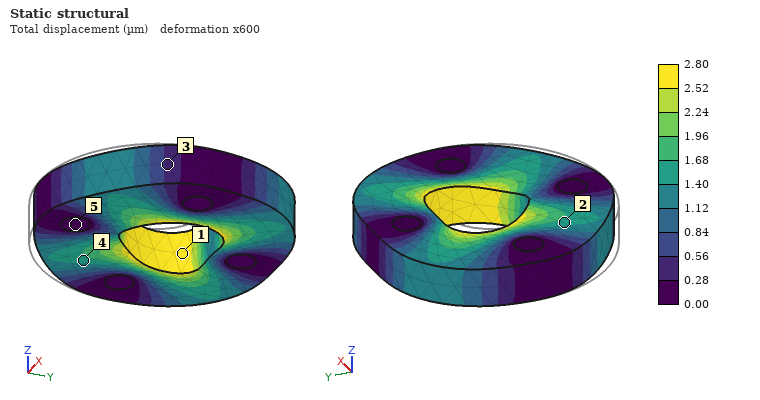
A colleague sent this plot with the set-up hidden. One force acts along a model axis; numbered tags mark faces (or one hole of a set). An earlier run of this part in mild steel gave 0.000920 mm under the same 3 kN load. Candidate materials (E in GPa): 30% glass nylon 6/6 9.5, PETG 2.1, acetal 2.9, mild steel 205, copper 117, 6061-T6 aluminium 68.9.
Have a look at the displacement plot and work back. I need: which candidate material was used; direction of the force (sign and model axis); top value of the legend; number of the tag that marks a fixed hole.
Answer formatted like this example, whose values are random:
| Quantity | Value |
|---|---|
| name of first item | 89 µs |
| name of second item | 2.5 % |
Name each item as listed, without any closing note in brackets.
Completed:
| Quantity | Value |
|---|---|
| which candidate material was used | 6061-T6 aluminium |
| direction of the force | +Y |
| top value of the legend | 2.80 µm |
| number of the tag that marks a fixed hole | 5 |
